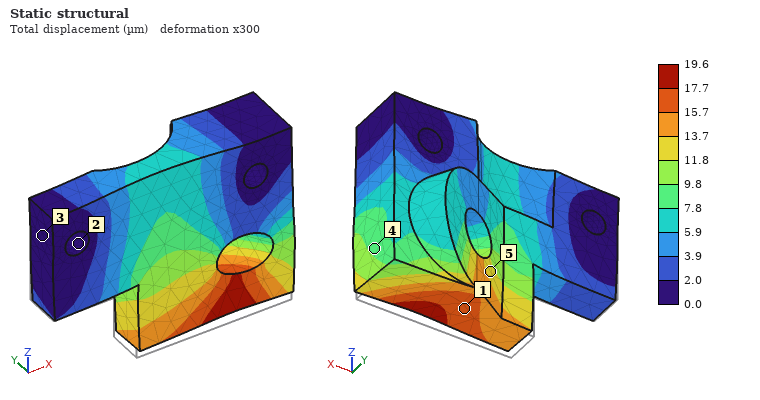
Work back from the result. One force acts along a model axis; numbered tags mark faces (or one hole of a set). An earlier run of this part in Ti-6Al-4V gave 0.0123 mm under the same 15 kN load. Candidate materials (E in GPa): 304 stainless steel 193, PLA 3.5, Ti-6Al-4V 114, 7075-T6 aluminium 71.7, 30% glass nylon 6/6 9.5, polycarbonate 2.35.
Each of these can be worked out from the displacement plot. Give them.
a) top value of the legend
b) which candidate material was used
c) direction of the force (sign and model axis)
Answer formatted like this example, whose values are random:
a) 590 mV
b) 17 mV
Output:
a) 19.6 µm
b) 7075-T6 aluminium
c) +Z
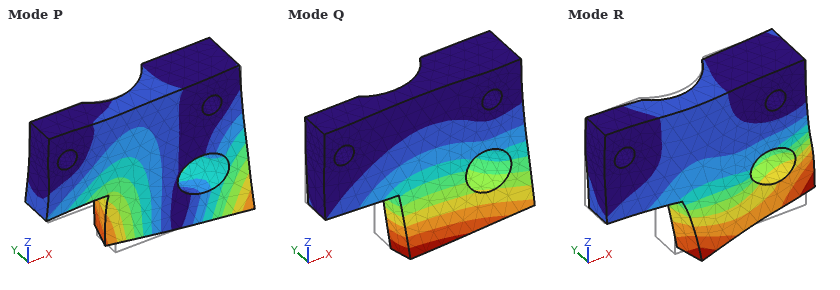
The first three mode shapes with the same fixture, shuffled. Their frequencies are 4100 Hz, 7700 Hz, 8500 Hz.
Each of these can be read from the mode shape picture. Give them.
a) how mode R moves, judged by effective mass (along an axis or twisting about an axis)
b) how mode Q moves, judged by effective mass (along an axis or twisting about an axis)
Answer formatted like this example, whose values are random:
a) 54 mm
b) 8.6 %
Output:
a) along X
b) along Y
